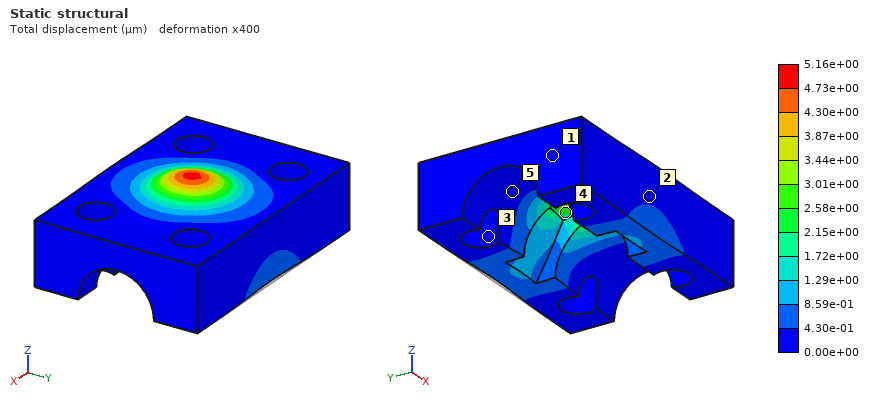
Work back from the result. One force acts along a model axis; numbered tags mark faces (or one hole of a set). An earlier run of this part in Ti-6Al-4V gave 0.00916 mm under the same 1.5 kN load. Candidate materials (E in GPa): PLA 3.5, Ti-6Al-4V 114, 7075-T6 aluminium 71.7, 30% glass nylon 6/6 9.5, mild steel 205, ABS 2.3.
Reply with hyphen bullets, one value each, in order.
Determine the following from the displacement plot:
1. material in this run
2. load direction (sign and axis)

- mild steel
- +Z
